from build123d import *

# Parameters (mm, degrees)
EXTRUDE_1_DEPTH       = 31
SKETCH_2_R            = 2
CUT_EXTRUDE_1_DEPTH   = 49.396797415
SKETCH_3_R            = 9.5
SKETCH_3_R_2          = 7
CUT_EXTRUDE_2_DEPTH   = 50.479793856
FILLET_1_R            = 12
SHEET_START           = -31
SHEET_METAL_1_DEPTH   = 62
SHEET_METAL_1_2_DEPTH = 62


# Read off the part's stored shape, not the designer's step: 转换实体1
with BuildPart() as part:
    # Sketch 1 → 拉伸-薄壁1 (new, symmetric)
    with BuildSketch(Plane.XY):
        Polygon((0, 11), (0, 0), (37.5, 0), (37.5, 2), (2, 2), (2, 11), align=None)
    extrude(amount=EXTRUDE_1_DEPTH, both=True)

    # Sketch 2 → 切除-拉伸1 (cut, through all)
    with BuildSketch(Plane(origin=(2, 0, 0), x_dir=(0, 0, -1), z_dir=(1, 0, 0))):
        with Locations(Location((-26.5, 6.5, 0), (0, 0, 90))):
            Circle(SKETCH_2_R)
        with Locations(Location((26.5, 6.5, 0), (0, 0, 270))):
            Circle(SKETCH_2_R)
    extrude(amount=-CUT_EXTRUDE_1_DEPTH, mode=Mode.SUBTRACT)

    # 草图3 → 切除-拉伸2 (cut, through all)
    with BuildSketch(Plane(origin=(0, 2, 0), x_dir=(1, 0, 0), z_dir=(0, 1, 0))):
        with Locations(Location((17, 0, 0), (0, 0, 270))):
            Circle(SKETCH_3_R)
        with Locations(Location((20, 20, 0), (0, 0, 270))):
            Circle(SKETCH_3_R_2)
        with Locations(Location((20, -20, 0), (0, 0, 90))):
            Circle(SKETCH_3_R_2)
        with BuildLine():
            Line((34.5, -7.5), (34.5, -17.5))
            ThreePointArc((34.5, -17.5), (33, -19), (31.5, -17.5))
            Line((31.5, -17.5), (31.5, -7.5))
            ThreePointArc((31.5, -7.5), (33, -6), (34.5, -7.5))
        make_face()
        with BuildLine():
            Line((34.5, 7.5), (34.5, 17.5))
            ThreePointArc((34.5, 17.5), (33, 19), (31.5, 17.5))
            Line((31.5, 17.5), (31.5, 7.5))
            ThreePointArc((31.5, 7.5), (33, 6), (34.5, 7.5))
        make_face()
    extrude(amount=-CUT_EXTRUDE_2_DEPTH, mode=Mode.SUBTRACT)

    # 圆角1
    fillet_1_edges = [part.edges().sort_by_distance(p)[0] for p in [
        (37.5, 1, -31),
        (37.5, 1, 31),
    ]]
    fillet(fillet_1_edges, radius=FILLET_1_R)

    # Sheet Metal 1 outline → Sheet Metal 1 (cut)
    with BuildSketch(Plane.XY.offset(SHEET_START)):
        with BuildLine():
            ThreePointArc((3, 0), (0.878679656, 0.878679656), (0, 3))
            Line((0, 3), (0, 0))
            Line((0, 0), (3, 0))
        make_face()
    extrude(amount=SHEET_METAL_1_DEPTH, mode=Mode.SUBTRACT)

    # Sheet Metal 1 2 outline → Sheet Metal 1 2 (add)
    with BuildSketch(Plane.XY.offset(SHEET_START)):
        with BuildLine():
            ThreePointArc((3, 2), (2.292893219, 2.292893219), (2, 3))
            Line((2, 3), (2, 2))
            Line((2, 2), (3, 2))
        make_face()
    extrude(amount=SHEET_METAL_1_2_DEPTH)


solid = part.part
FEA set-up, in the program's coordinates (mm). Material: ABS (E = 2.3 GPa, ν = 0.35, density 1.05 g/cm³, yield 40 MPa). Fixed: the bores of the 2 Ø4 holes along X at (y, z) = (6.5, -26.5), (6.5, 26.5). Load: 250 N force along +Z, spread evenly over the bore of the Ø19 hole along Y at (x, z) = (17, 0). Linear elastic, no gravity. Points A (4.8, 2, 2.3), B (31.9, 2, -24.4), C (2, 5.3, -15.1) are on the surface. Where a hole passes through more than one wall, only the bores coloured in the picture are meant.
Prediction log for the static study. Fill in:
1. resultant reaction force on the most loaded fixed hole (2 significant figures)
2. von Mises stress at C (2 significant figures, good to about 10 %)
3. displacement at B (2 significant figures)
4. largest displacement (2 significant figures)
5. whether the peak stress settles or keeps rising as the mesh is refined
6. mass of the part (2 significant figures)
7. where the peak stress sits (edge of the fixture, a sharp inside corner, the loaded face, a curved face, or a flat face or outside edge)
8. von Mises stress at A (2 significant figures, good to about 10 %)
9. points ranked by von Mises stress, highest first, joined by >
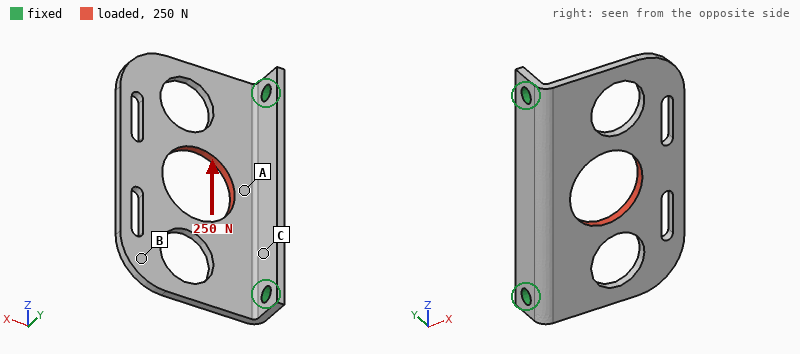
150 N
5.5 MPa
0.59 mm
0.66 mm
keeps rising
4.4 g
edge of the fixture
9.6 MPa
A > C > B
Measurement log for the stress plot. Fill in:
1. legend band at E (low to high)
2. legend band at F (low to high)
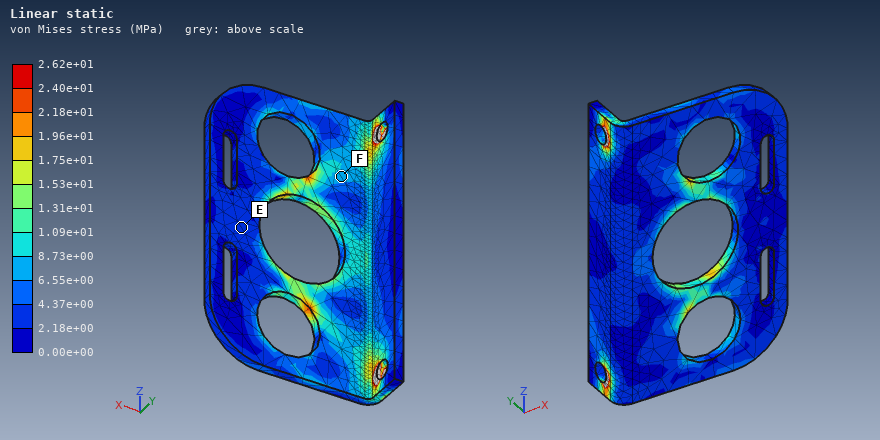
2.18e+00 to 4.37e+00 MPa
6.55e+00 to 8.73e+00 MPa
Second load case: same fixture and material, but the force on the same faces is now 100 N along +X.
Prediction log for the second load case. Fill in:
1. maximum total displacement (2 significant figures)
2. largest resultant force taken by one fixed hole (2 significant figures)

0.87 mm
54 N
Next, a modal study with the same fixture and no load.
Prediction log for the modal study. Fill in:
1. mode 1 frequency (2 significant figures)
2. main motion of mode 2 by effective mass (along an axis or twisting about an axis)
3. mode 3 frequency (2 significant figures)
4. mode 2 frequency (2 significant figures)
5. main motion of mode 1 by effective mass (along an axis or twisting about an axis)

270 Hz
twisting about X
1200 Hz
570 Hz
along Y
